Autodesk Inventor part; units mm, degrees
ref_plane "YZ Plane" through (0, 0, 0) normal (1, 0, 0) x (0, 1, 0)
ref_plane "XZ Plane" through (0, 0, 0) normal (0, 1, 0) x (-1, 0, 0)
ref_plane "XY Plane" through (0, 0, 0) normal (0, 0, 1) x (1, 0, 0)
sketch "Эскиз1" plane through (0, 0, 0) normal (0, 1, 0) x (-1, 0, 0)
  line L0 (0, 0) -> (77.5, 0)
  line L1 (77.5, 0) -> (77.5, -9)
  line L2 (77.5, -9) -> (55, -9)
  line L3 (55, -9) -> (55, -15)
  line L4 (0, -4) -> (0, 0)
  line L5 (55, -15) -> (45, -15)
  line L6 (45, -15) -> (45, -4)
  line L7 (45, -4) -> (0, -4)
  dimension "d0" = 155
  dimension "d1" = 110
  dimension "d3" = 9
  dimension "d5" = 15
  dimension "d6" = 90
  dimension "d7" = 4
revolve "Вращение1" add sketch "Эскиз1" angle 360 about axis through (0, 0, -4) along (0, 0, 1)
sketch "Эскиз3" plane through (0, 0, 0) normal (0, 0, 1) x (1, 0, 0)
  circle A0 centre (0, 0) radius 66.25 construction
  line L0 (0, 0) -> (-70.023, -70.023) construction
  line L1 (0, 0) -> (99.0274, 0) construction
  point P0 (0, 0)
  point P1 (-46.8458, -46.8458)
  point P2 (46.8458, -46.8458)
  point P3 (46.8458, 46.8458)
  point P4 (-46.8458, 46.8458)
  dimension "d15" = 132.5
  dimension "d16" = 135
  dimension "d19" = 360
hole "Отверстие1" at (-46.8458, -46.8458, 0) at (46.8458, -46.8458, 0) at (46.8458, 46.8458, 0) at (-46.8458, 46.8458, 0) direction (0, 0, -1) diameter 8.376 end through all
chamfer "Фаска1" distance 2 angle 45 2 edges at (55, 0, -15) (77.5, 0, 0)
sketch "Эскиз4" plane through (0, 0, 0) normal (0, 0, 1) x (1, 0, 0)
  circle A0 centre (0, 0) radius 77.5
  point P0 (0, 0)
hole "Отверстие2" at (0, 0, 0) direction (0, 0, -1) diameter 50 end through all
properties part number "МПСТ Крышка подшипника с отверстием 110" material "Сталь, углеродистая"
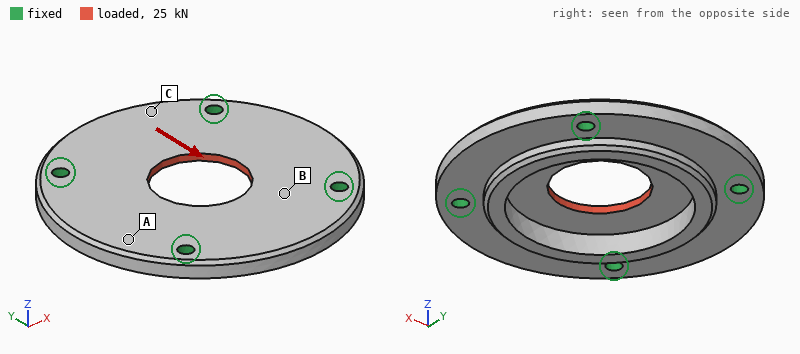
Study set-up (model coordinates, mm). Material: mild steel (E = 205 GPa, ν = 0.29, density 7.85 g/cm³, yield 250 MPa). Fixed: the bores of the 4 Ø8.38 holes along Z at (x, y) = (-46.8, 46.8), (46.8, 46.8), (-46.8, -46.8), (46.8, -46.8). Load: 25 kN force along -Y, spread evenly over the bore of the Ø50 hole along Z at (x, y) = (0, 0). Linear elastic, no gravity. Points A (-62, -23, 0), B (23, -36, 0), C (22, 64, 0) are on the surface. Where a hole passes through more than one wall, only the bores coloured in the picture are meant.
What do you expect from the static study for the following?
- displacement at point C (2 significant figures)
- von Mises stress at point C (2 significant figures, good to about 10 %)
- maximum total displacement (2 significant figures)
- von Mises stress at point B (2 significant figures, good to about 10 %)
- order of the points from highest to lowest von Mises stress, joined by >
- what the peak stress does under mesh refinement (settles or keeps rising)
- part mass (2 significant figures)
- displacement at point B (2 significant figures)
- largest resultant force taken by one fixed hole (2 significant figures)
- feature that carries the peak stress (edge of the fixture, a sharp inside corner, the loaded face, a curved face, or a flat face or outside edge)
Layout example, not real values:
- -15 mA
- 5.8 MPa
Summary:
- 6.4 µm
- 15 MPa
- 15 µm
- 33 MPa
- B > C > A
- keeps rising
- 1.1 kg
- 7.4 µm
- 6.3 kN
- edge of the fixture
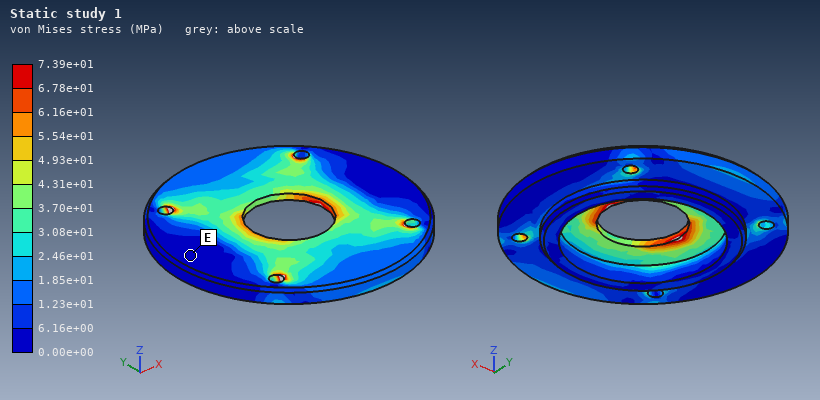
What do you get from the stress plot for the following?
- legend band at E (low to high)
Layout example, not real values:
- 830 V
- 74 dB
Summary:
- 0.00e+00 to 6.16e+00 MPa
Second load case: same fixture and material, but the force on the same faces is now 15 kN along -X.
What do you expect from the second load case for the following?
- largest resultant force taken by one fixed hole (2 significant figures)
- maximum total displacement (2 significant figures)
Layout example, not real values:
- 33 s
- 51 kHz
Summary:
- 3.8 kN
- 8.8 µm
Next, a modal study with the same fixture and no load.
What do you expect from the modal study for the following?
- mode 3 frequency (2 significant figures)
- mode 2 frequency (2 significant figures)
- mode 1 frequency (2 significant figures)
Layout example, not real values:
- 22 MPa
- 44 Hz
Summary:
- 4900 Hz
- 4900 Hz
- 4300 Hz
